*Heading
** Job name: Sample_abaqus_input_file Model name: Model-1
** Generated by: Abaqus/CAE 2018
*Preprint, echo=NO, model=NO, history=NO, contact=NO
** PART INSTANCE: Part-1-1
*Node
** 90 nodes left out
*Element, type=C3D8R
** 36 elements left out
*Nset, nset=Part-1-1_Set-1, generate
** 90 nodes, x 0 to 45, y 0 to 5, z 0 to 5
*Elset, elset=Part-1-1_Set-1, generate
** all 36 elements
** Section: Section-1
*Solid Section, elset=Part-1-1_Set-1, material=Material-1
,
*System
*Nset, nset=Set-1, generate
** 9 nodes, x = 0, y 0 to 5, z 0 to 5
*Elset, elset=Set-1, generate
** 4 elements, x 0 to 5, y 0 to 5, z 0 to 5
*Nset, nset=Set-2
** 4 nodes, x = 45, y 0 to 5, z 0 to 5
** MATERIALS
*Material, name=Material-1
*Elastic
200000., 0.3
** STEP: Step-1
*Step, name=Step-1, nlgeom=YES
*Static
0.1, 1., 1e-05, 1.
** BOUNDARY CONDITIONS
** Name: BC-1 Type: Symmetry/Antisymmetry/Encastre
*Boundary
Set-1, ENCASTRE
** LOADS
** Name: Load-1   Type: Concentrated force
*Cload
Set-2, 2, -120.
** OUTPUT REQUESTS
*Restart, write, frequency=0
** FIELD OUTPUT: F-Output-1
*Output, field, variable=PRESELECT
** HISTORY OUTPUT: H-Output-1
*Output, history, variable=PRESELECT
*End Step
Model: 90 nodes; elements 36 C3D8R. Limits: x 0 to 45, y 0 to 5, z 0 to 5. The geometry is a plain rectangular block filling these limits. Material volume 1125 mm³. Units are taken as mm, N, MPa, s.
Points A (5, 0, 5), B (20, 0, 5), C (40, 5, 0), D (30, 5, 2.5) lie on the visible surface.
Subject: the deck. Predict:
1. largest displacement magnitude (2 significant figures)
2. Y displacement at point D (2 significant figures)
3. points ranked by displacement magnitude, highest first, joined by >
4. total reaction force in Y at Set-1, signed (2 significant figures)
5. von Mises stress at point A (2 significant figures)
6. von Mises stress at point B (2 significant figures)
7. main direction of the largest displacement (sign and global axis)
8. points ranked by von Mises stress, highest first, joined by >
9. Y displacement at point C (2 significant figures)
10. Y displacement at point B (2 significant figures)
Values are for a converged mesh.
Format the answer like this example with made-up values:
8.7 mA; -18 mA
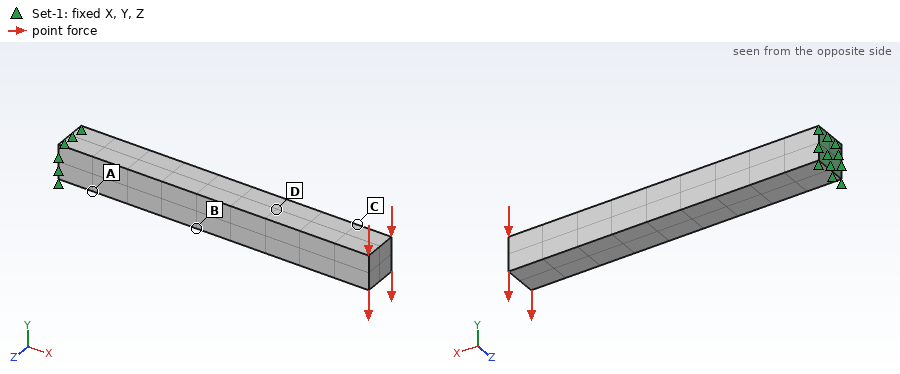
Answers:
1.4 mm; -0.73 mm; C > D > B > A; 480 N; 900 MPa; 570 MPa; -Y; A > B > D > C; -1.2 mm; -0.35 mm
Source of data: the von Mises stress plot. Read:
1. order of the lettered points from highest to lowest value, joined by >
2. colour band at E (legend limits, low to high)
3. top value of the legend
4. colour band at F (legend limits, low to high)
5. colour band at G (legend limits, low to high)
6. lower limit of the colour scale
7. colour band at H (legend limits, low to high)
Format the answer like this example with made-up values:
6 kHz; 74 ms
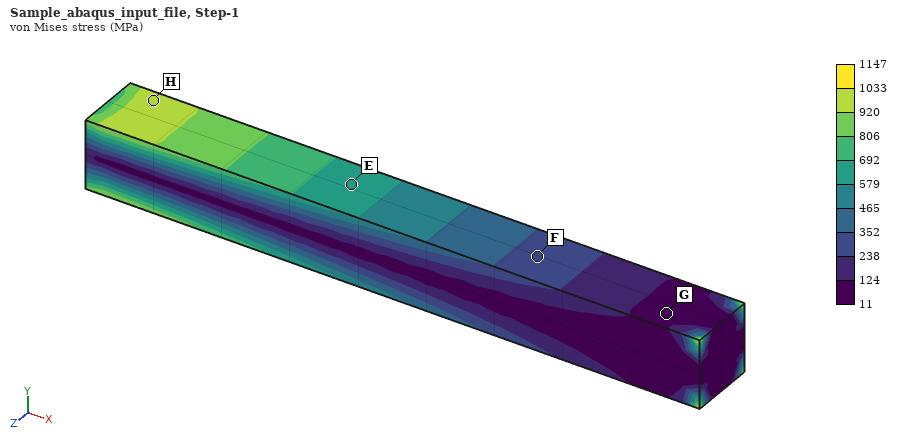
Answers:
H > E > F > G; 579 to 692 MPa; 1147 MPa; 238 to 352 MPa; 11 to 124 MPa; 11 MPa; 920 to 1033 MPa
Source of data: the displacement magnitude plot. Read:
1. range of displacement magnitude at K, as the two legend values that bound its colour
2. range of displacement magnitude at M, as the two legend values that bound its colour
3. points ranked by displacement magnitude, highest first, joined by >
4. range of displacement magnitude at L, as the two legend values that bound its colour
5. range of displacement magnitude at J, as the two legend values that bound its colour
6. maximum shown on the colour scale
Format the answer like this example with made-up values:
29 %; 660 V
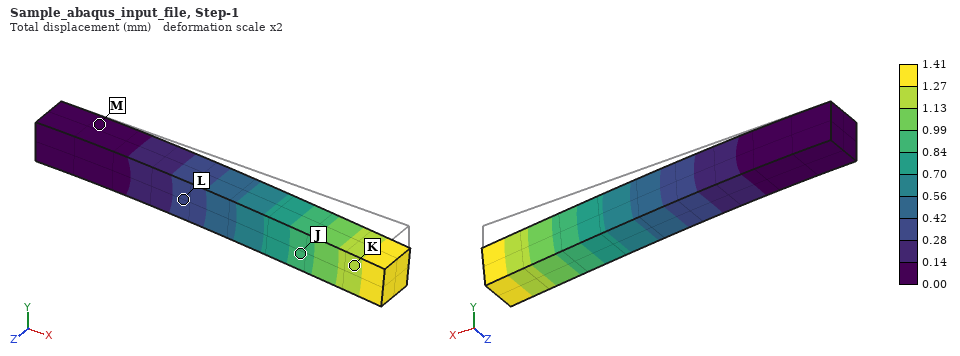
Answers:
1.13 to 1.27 mm; 0.00 to 0.14 mm; K > J > L > M; 0.28 to 0.42 mm; 0.84 to 0.99 mm; 1.41 mm
